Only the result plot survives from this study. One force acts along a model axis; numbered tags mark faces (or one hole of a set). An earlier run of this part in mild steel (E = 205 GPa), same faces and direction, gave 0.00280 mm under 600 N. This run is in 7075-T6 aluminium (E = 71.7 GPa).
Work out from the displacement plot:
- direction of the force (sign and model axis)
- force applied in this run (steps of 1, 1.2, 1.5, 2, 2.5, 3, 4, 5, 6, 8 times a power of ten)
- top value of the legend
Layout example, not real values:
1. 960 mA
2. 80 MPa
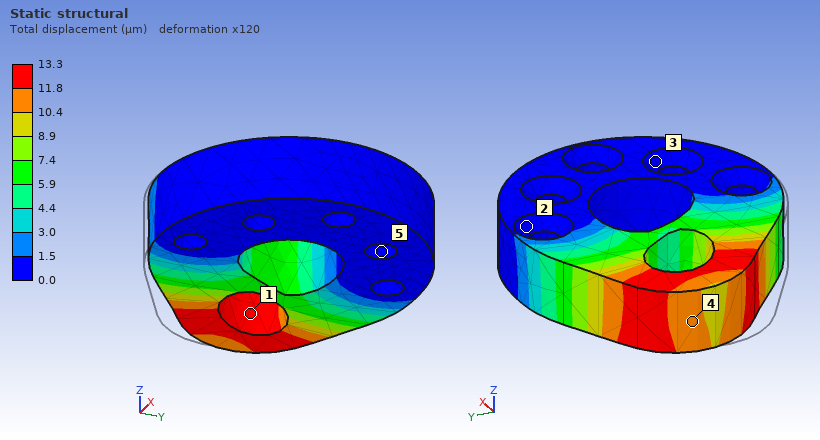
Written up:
1. +Y
2. 1 kN
3. 13.3 µm
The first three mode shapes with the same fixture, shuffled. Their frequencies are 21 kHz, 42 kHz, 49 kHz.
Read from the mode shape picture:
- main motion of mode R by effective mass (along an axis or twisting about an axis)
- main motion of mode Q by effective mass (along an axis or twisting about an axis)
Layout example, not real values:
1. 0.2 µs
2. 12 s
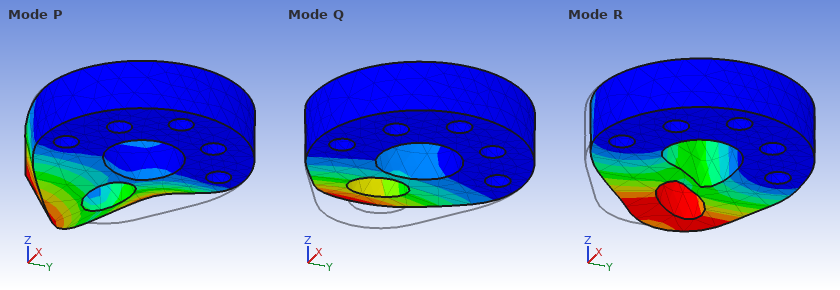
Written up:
1. along Y
2. along Z
